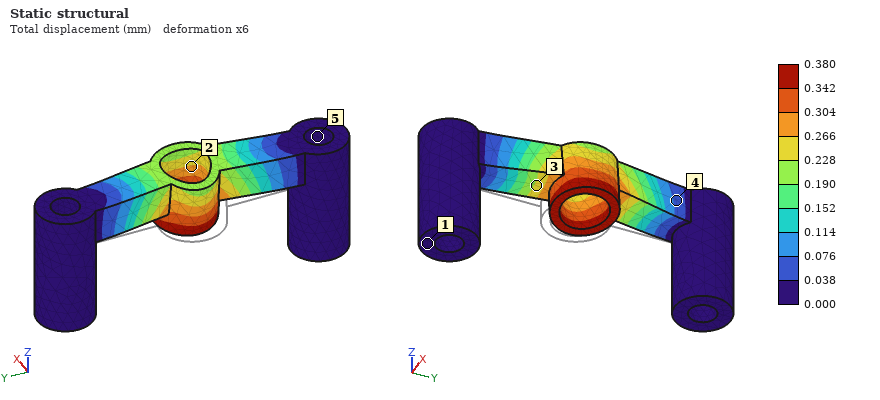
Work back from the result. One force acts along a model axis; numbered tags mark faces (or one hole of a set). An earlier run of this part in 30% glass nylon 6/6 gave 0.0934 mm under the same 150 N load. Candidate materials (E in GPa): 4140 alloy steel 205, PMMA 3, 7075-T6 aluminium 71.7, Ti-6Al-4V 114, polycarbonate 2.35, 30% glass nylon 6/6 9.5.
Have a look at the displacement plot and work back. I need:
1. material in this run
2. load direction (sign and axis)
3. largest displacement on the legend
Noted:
polycarbonate
+X
0.380 mm
